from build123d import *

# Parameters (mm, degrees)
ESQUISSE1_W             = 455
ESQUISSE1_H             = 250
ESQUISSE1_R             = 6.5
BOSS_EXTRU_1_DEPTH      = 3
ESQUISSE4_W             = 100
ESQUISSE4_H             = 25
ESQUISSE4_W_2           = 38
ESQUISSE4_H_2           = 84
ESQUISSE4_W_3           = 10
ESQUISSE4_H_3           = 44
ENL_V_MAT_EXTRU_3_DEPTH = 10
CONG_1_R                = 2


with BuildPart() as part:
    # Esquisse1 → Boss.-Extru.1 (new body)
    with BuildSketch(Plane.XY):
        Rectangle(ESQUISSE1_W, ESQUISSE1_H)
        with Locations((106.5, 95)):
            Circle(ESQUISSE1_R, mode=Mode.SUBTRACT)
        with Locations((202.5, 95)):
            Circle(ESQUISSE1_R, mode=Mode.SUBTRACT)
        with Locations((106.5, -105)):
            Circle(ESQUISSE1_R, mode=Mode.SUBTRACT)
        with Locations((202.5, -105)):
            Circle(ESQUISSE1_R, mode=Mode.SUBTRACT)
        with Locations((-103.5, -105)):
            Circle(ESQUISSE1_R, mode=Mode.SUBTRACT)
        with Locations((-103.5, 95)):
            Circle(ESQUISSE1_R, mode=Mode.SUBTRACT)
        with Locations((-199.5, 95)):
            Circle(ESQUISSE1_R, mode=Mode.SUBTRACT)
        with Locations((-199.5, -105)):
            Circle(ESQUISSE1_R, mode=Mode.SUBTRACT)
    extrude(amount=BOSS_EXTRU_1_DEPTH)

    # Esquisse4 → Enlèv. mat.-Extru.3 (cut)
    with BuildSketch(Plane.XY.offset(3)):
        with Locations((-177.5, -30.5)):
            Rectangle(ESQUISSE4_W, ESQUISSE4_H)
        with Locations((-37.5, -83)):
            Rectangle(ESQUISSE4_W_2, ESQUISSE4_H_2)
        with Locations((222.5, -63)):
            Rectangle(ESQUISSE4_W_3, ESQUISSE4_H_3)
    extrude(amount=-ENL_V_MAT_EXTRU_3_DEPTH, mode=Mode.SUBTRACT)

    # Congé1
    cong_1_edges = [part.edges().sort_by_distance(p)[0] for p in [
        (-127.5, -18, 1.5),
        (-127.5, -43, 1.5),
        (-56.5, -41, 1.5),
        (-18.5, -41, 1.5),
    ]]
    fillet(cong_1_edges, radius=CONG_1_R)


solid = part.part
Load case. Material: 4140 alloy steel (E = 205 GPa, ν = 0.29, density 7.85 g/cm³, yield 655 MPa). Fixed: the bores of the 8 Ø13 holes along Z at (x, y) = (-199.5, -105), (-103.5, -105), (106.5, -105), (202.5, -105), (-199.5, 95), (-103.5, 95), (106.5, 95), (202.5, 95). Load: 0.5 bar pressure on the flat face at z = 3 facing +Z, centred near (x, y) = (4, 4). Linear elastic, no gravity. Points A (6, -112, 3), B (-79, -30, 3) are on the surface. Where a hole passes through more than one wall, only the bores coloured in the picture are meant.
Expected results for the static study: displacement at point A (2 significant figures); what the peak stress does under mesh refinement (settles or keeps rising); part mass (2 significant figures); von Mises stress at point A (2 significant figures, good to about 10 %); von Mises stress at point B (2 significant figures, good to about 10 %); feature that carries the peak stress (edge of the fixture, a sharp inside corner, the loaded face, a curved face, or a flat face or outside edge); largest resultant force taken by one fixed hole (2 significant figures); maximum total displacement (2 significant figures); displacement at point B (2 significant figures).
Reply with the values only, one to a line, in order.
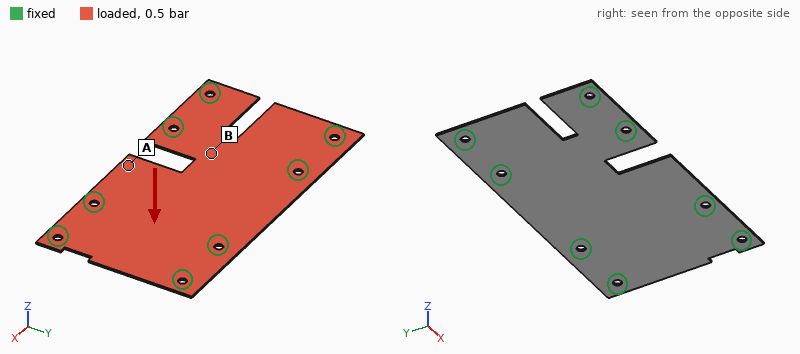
1.2 mm
keeps rising
2.5 kg
34 MPa
94 MPa
edge of the fixture
1.0 kN
1.5 mm
0.79 mm
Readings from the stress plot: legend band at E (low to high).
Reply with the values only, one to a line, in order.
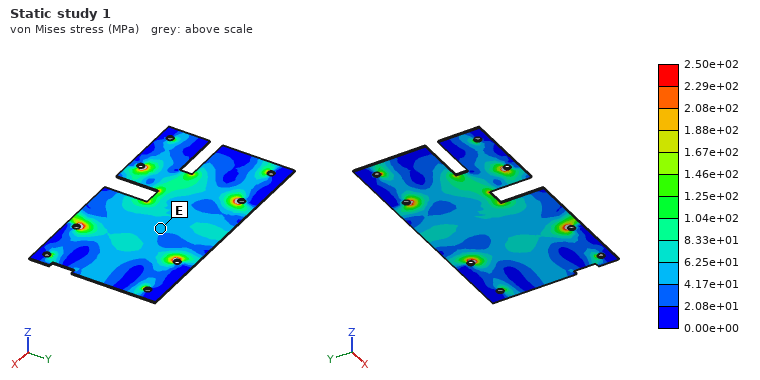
4.17e+01 to 6.25e+01 MPa
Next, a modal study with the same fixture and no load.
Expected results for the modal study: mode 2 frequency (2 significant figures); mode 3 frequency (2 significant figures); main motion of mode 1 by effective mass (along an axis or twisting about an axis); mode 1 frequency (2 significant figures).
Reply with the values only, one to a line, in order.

320 Hz
360 Hz
along Z
250 Hz
